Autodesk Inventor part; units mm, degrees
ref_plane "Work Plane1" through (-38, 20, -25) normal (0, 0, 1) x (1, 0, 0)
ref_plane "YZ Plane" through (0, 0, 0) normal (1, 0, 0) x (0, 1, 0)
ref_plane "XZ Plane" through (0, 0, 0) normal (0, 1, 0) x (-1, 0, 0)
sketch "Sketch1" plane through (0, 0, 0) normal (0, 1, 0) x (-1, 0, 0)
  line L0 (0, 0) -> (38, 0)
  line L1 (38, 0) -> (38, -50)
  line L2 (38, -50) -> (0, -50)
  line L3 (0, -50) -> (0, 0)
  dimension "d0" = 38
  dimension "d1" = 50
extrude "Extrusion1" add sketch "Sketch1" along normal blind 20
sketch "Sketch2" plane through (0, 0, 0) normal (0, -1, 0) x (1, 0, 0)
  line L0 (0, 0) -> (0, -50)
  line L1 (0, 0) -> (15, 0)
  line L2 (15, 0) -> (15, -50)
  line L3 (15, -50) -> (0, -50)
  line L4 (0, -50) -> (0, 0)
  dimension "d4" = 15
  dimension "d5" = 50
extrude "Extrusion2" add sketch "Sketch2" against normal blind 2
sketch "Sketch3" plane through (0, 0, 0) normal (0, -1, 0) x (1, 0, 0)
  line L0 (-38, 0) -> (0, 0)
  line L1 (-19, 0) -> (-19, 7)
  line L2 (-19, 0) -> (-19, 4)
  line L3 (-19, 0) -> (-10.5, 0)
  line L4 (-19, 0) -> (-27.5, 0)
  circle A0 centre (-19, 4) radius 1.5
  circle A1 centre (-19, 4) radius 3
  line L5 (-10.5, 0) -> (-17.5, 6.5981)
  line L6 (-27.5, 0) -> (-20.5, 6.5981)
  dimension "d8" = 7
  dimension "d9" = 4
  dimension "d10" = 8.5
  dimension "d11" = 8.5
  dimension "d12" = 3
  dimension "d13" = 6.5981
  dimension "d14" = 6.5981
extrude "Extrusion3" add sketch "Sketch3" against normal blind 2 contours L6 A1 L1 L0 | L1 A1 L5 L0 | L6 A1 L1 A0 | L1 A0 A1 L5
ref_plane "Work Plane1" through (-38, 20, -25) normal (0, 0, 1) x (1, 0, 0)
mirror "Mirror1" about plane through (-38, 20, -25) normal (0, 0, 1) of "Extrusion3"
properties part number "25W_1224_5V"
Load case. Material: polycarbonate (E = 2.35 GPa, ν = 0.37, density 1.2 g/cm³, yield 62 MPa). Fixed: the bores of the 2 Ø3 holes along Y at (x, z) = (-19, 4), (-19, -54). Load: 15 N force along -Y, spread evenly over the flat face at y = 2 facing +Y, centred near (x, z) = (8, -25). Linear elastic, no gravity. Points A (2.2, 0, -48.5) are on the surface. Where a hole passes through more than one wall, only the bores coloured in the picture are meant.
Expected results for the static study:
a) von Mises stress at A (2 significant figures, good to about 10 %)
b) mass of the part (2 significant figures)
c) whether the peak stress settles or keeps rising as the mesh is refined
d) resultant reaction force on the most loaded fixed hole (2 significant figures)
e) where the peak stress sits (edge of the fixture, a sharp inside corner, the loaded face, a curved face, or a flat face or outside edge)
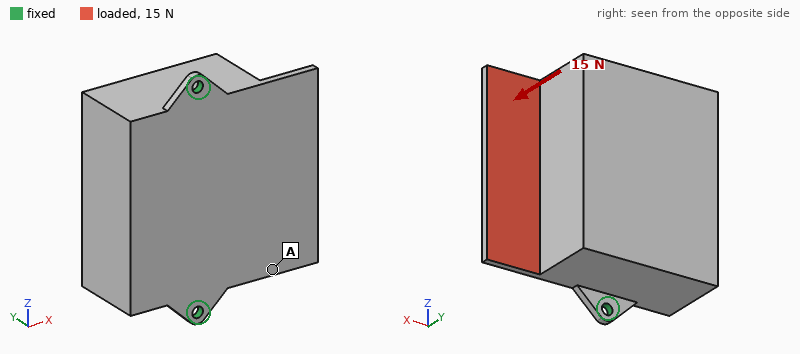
2.2 MPa
48 g
keeps rising
8.9 N
edge of the fixture
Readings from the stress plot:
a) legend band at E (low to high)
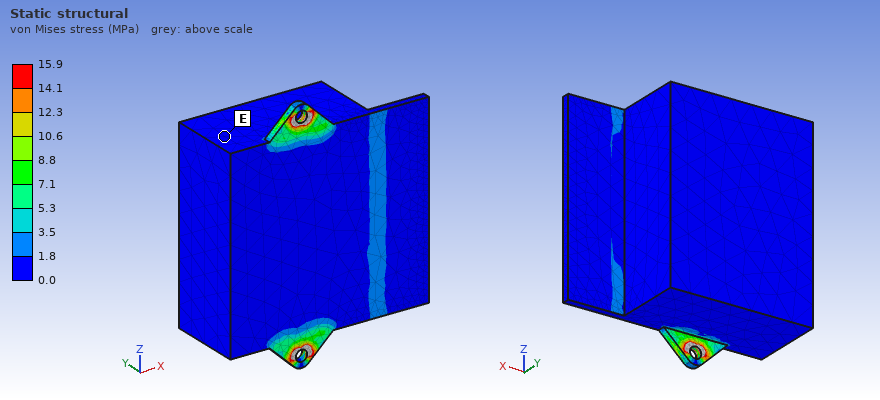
0.0 to 1.8 MPa
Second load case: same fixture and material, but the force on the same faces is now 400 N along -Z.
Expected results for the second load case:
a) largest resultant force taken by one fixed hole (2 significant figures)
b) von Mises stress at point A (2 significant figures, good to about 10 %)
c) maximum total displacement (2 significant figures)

270 N
7.4 MPa
0.29 mm
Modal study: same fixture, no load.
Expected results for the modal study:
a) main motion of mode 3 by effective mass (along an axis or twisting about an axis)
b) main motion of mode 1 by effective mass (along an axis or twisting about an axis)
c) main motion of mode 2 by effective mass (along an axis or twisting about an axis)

along Z
along X
along Y
